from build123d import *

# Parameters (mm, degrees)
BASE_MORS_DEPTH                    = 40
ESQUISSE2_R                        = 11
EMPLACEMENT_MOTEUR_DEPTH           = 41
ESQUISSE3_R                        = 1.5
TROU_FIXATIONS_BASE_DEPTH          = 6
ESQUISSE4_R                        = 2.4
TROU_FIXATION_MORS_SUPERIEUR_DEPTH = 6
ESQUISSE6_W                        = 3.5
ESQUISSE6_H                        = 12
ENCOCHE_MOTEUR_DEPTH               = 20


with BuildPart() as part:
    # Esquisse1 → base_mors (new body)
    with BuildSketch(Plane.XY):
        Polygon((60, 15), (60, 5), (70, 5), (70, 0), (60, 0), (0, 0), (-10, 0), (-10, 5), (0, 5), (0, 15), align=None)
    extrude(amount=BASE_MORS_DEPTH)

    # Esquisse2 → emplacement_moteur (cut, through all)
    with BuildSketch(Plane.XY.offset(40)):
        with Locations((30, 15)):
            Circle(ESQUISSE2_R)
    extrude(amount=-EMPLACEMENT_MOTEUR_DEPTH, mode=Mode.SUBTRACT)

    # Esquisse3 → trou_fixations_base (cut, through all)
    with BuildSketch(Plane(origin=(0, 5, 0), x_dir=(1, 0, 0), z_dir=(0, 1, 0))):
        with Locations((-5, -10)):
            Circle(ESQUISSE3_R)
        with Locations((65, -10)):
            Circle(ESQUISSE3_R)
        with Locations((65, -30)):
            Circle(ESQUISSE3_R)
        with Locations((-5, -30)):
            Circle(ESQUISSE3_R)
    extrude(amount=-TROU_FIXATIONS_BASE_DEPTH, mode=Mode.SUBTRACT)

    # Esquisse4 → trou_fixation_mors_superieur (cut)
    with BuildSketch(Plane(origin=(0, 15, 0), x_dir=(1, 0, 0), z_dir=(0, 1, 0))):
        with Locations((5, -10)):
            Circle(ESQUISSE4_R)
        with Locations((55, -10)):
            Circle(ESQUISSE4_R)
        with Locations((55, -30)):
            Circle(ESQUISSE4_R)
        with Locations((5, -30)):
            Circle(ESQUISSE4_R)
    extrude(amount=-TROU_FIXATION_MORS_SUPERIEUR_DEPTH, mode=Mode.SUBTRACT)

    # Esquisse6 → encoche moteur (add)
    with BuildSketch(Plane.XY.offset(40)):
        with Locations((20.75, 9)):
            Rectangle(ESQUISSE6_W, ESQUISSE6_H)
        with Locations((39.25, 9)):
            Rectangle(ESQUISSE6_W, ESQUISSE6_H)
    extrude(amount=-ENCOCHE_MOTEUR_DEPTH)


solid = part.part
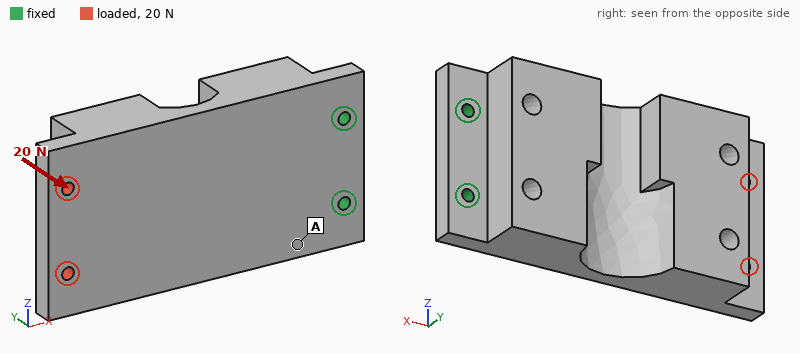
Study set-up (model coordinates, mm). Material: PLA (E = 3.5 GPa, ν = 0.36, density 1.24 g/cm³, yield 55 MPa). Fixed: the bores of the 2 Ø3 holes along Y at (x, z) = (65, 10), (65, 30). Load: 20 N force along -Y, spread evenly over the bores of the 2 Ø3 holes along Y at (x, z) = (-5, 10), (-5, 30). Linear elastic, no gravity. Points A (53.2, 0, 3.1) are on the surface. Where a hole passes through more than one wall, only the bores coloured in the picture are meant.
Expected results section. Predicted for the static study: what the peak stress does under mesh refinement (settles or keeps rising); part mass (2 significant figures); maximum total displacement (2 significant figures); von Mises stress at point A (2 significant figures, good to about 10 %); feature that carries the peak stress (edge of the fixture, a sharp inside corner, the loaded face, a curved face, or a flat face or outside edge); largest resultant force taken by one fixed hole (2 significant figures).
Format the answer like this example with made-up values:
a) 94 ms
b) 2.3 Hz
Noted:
a) keeps rising
b) 40 g
c) 1.0 mm
d) 1.5 MPa
e) edge of the fixture
f) 10 N
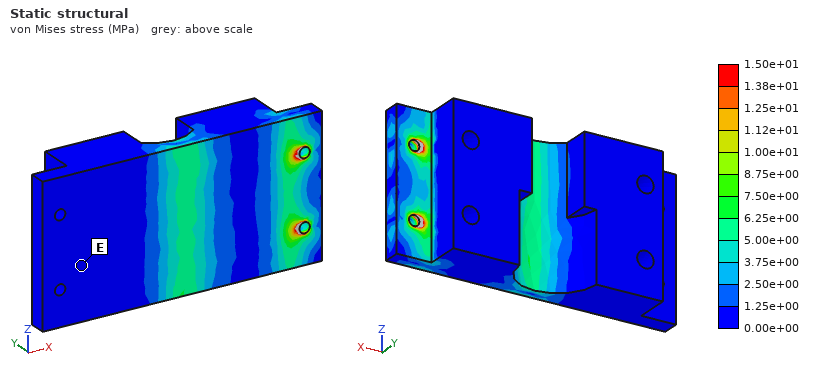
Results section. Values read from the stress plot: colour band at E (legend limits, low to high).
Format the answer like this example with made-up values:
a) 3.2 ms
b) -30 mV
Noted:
a) 0.00e+00 to 1.25e+00 MPa
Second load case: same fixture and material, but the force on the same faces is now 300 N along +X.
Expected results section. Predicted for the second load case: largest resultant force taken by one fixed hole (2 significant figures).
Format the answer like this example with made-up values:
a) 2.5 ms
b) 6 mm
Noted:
a) 150 N
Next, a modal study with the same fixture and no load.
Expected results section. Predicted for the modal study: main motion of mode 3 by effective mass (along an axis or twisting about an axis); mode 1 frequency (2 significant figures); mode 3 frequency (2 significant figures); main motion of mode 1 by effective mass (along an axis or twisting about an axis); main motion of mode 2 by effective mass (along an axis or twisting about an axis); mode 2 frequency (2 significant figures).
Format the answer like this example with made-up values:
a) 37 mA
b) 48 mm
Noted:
a) along Y
b) 220 Hz
c) 1200 Hz
d) along Y
e) along Z
f) 970 Hz
